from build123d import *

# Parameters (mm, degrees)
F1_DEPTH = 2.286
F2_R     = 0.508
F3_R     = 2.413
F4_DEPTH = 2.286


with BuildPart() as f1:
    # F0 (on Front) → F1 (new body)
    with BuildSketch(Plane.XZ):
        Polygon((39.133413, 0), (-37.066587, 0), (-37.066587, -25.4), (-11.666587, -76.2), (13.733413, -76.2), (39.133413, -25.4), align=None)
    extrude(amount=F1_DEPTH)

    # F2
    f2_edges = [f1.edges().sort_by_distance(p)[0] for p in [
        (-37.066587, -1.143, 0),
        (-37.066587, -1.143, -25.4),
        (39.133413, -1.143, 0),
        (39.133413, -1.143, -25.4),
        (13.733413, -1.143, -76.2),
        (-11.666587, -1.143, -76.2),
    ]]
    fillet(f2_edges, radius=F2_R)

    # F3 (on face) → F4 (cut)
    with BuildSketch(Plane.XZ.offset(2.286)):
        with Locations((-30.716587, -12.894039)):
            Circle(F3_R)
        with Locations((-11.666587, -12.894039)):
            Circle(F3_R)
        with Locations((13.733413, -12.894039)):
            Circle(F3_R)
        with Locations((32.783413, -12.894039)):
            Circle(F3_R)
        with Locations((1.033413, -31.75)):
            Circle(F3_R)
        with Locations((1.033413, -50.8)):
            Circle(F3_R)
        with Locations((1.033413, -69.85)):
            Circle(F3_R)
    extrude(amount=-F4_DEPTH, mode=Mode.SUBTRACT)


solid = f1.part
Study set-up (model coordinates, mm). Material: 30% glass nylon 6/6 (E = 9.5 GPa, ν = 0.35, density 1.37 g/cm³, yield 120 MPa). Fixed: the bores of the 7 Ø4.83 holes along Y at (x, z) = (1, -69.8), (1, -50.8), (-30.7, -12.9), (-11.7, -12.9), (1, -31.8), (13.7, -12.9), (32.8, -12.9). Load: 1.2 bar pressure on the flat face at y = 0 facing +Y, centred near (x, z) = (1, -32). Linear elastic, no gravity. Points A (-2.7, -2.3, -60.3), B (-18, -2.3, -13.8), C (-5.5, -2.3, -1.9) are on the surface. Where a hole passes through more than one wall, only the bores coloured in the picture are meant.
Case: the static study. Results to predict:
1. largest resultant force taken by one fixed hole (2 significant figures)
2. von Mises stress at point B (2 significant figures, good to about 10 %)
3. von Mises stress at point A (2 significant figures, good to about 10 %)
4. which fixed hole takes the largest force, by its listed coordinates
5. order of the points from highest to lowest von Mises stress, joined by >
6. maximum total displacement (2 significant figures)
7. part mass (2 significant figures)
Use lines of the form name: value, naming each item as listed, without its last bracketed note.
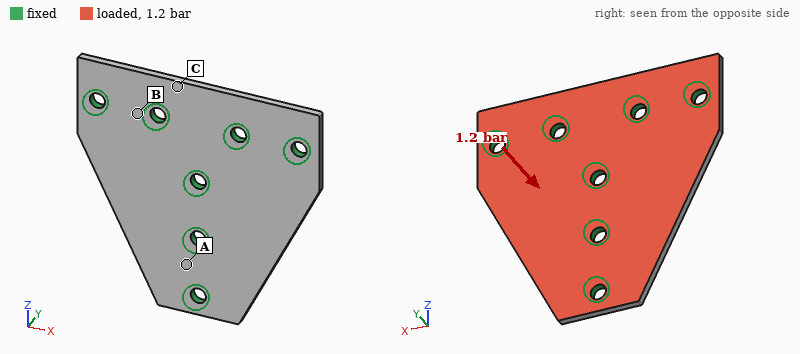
largest resultant force taken by one fixed hole: 120 N
von Mises stress at point B: 8.4 MPa
von Mises stress at point A: 15 MPa
which fixed hole takes the largest force, by its listed coordinates: (1, -50.8)
order of the points from highest to lowest von Mises stress, joined by >: A > B > C
maximum total displacement: 0.34 mm
part mass: 14 g
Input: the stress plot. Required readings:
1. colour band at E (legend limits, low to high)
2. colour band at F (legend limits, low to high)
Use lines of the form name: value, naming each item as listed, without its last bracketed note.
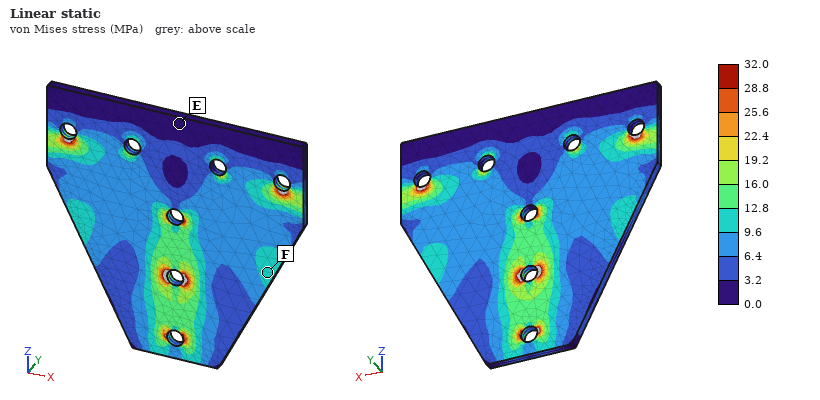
colour band at E: 0.0 to 3.2 MPa
colour band at F: 9.6 to 12.8 MPa
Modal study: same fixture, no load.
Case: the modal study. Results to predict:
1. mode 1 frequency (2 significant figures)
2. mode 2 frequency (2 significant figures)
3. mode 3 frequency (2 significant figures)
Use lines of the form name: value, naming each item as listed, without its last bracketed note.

mode 1 frequency: 2300 Hz
mode 2 frequency: 2300 Hz
mode 3 frequency: 4400 Hz
